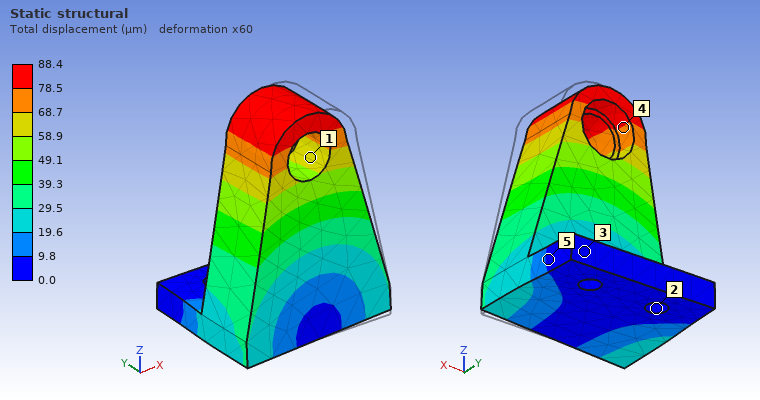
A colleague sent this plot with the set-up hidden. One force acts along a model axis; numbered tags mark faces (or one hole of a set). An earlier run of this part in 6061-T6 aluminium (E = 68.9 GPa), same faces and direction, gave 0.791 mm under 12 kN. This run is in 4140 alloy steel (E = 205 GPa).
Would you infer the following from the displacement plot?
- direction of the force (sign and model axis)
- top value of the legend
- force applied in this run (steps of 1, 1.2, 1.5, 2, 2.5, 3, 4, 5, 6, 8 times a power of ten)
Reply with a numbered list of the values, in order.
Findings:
1. -X
2. 88.4 µm
3. 4 kN
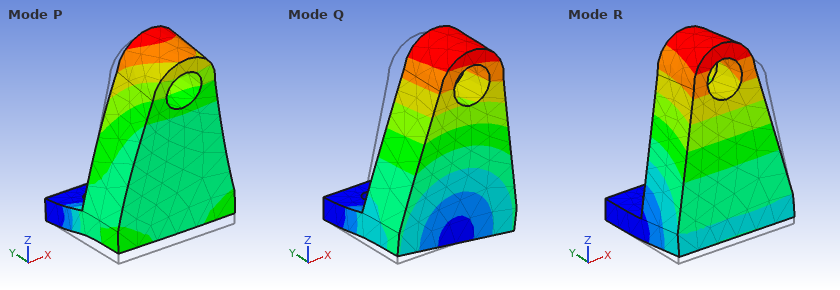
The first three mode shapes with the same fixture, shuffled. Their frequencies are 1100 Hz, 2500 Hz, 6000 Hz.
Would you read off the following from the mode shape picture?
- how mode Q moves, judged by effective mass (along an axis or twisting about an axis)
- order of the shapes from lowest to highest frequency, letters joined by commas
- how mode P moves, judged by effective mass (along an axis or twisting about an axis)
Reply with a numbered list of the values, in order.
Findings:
1. along X
2. R, Q, P
3. along Z
